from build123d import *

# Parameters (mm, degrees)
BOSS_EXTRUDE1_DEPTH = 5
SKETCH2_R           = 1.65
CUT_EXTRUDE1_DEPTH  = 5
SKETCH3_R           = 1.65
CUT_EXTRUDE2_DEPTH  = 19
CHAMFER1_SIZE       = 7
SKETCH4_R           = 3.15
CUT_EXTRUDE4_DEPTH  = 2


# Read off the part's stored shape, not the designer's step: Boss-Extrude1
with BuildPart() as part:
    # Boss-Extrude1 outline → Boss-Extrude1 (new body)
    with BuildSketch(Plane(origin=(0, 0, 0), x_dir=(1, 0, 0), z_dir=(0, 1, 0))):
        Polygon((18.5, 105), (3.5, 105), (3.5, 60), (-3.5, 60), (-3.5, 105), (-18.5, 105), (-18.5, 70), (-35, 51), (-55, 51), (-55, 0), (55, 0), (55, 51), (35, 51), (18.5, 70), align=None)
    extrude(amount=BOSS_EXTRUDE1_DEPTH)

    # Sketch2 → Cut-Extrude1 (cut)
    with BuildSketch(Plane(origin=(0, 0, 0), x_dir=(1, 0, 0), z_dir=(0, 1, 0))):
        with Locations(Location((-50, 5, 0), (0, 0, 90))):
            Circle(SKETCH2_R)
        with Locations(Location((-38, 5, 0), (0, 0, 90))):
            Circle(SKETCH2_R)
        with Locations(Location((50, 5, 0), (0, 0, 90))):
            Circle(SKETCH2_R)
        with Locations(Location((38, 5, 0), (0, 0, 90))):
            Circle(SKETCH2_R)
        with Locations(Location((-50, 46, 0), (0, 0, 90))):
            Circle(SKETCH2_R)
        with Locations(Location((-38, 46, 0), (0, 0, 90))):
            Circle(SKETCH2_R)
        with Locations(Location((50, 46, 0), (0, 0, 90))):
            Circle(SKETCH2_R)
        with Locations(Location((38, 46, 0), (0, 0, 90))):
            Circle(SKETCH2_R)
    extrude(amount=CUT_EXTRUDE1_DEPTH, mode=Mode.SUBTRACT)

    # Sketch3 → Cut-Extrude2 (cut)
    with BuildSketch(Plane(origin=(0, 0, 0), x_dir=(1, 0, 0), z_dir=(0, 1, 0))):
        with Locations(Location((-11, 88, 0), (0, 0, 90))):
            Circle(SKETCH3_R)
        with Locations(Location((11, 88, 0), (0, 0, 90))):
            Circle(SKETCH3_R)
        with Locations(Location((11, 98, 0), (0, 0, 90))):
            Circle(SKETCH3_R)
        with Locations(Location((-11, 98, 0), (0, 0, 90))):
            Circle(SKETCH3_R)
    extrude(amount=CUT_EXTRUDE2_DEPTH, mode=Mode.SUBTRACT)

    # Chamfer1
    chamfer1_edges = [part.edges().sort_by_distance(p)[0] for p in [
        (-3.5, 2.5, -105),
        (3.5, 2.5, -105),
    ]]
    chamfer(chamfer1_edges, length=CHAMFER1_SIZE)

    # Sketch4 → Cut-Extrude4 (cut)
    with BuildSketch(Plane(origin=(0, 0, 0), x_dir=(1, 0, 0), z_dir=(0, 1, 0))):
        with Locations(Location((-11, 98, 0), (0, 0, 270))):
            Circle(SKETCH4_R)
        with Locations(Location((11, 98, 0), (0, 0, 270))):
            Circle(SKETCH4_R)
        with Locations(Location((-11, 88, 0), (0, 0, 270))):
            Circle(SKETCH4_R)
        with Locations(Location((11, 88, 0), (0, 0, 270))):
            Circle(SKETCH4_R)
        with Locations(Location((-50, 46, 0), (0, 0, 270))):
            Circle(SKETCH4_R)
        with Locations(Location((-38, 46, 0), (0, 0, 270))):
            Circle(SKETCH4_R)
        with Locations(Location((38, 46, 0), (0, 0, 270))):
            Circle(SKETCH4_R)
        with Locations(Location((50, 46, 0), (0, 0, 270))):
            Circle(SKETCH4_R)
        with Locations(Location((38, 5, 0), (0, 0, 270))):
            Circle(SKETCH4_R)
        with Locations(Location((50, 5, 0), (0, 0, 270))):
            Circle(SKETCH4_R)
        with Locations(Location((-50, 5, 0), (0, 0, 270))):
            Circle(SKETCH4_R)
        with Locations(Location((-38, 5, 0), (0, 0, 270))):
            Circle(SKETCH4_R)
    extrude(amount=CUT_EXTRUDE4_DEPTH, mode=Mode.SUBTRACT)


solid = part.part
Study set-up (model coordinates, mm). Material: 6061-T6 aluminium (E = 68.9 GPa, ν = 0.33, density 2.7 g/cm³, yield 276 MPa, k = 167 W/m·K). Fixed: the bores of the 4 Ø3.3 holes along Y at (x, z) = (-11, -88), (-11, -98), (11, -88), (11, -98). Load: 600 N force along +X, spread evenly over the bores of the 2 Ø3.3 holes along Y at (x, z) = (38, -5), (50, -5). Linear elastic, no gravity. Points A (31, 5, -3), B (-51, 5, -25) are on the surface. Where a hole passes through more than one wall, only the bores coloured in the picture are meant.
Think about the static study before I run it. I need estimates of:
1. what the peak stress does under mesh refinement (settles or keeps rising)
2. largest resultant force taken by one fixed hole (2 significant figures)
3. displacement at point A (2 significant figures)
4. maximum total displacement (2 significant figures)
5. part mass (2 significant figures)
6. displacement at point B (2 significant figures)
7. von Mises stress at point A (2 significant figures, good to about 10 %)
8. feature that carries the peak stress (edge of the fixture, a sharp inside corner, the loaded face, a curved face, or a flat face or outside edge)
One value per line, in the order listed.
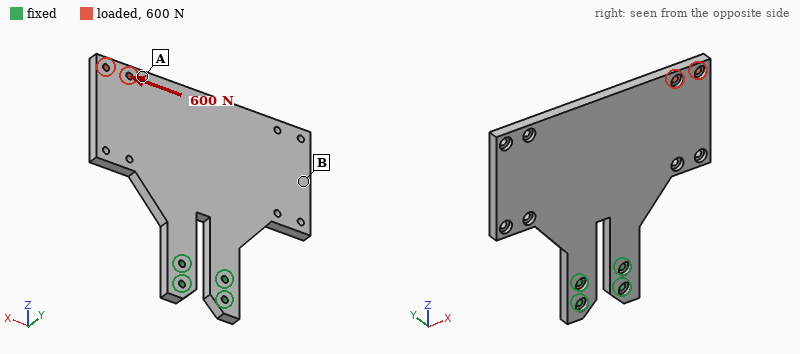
keeps rising
1.5 kN
0.13 mm
0.17 mm
99 g
0.12 mm
14 MPa
edge of the fixture
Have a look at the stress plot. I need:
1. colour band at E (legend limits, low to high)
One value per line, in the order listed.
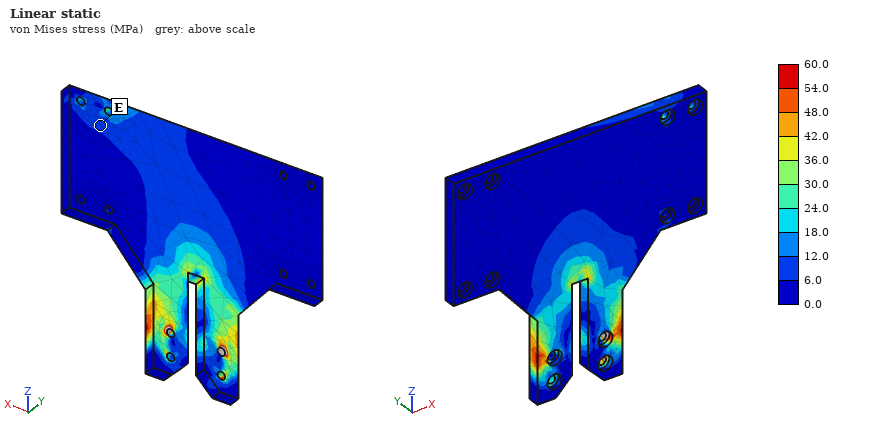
6.0 to 12.0 MPa
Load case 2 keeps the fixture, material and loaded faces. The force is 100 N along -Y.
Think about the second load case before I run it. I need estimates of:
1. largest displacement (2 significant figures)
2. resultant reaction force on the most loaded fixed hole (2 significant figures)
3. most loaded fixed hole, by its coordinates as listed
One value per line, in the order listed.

1.3 mm
520 N
(11, -88)
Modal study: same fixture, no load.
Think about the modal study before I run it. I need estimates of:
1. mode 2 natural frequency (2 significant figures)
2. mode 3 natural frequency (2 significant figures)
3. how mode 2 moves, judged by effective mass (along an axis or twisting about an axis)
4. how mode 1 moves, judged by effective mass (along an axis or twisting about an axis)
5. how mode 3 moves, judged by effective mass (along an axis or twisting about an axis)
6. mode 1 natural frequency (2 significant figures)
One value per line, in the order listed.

540 Hz
1500 Hz
twisting about Z
along Y
along X
280 Hz
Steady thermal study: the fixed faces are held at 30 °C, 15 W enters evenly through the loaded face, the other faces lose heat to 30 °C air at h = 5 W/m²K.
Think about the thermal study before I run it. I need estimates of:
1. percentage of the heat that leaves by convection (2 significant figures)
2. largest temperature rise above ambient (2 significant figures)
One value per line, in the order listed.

12 %
45 K
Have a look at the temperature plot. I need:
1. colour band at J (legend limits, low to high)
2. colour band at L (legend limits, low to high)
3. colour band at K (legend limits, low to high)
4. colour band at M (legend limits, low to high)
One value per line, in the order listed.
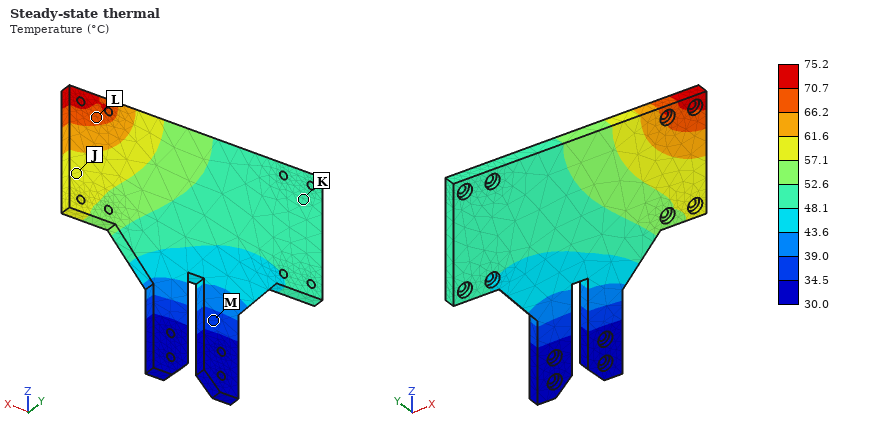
57.1 to 61.6 °C
66.2 to 70.7 °C
48.1 to 52.6 °C
34.5 to 39.0 °C
